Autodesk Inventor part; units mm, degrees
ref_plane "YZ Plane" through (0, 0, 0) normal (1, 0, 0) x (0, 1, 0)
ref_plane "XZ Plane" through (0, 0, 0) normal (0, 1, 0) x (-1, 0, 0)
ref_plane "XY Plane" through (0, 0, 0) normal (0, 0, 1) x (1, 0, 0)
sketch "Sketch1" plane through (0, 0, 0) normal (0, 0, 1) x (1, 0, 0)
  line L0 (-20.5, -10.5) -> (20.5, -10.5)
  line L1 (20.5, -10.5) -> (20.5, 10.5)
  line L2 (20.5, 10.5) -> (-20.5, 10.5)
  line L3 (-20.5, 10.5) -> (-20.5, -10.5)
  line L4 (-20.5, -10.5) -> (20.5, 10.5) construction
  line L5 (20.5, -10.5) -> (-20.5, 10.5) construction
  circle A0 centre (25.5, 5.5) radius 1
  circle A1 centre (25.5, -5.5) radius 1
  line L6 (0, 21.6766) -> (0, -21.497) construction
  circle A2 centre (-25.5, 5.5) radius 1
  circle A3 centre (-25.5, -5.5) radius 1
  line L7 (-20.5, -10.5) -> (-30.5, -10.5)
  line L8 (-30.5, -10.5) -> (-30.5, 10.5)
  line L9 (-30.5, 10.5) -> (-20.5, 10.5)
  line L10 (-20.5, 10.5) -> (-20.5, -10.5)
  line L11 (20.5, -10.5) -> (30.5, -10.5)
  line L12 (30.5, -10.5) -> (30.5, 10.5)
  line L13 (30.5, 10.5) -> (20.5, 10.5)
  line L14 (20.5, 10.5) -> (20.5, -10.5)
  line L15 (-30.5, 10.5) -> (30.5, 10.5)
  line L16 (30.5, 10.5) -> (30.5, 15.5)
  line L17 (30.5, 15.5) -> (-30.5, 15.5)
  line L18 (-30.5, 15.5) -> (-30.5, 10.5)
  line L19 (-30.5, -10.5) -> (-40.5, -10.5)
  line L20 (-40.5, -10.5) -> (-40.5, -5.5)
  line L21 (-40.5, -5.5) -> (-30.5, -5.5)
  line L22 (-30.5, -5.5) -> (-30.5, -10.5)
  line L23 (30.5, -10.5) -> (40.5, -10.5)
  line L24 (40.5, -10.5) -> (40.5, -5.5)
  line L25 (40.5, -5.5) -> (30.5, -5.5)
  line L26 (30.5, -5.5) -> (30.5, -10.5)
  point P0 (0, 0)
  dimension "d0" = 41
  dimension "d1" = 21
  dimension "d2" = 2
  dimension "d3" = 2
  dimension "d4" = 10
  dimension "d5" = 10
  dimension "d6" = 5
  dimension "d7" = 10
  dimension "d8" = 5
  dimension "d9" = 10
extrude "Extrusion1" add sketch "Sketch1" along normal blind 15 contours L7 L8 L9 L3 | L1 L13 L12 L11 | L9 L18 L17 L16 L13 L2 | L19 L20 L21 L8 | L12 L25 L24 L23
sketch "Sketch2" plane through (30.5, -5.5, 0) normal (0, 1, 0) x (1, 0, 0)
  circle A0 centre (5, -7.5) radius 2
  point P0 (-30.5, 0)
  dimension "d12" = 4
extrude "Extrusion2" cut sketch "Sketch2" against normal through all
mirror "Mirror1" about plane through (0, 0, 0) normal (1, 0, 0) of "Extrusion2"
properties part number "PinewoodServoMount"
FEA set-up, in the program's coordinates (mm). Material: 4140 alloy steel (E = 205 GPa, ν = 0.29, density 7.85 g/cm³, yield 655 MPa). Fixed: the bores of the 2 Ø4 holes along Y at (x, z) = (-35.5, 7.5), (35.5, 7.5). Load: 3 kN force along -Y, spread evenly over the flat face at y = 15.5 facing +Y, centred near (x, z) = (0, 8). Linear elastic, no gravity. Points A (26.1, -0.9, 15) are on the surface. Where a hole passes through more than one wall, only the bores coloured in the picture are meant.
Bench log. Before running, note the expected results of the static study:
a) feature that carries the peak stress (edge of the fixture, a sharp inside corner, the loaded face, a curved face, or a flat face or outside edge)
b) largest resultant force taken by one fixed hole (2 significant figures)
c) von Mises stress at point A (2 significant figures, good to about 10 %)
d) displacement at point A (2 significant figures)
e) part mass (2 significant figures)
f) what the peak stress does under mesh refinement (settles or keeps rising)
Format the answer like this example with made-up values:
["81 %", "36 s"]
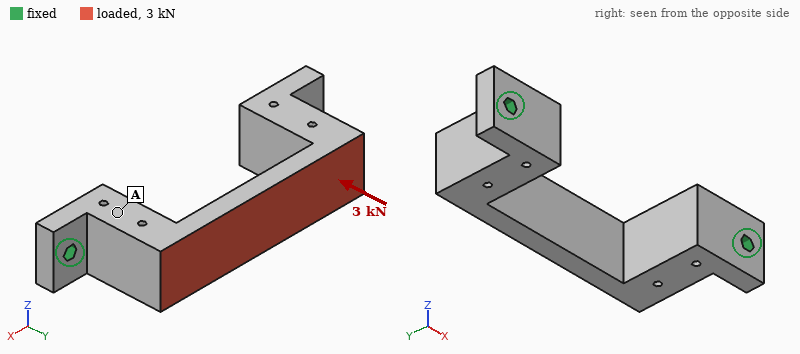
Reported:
["edge of the fixture", "1.8 kN", "22 MPa", "4.2 µm", "95 g", "keeps rising"]
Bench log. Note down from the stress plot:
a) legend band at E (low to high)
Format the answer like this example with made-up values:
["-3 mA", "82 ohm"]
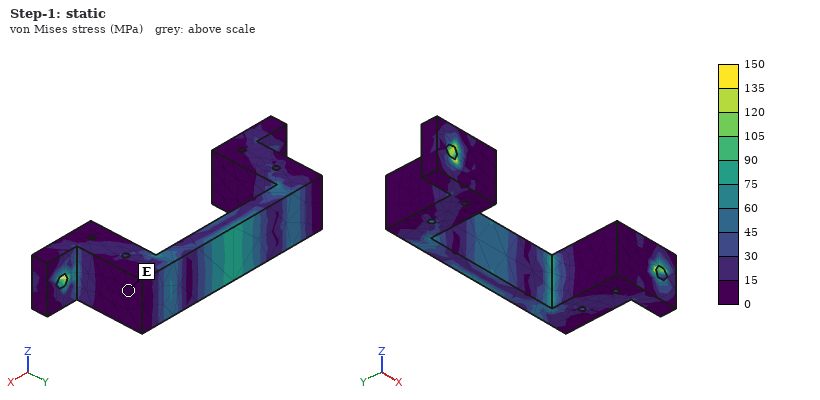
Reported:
["0 to 15 MPa"]
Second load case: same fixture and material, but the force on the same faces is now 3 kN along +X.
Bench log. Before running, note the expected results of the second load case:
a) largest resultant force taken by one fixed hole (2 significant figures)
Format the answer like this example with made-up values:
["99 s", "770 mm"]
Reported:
["1.7 kN"]
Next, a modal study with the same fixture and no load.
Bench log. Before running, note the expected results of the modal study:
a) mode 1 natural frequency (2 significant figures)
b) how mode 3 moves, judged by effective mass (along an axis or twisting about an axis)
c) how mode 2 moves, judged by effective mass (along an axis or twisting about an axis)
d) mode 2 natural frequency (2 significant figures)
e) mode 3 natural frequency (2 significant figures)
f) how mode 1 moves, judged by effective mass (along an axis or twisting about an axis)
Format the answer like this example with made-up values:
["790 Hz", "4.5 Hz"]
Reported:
["3800 Hz", "twisting about Y", "along X", "4800 Hz", "7000 Hz", "along Z"]
